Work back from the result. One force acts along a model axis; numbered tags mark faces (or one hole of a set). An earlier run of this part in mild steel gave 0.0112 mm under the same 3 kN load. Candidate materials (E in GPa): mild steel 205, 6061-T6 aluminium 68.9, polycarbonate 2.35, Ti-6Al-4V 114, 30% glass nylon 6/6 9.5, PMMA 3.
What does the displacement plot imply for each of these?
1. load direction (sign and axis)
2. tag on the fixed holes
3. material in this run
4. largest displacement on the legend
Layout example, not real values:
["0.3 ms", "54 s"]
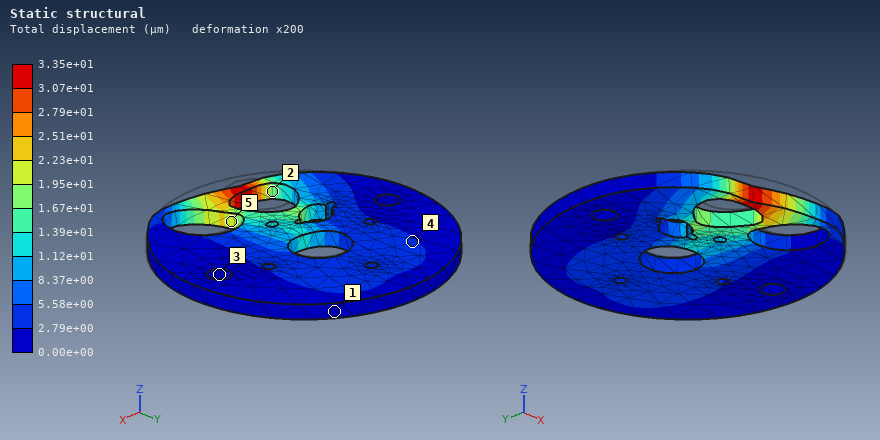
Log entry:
["+Y", "3", "6061-T6 aluminium", "3.35e+01 µm"]
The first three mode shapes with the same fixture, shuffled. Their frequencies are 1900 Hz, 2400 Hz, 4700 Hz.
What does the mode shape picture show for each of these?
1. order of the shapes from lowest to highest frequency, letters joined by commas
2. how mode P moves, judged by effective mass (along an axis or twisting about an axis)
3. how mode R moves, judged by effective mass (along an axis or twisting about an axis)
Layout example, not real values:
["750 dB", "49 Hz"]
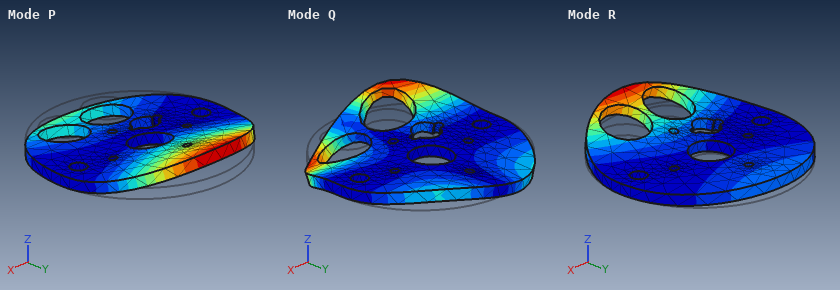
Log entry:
["P, R, Q", "along Z", "along Z"]
